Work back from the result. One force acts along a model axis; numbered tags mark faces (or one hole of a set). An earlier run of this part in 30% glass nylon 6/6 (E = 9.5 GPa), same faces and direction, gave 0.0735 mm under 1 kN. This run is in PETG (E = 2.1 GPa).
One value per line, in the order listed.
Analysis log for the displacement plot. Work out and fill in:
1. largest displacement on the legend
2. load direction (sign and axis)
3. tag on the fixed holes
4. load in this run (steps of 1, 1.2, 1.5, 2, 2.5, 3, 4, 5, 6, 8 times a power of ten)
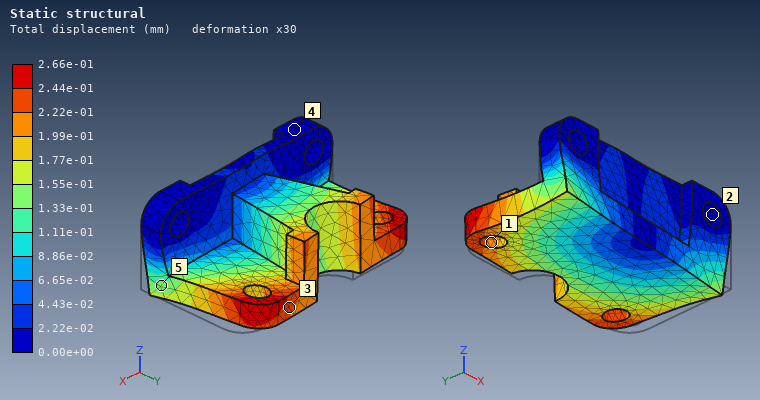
2.66e-01 mm
-X
2
800 N
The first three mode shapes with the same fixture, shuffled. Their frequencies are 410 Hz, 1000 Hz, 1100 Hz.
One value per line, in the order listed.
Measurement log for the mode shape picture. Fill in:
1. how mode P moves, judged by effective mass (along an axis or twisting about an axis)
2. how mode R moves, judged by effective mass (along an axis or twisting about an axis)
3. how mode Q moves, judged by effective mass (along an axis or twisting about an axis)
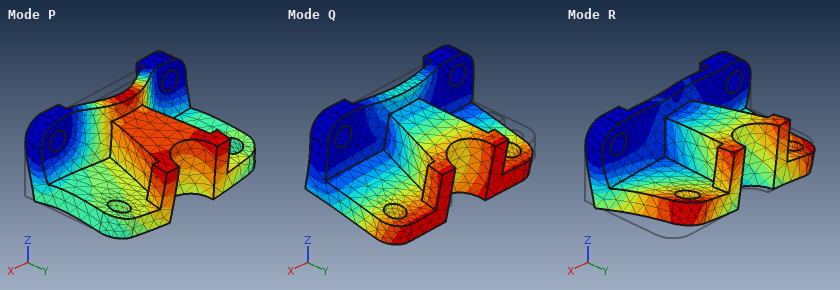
along Y
along X
along Z
